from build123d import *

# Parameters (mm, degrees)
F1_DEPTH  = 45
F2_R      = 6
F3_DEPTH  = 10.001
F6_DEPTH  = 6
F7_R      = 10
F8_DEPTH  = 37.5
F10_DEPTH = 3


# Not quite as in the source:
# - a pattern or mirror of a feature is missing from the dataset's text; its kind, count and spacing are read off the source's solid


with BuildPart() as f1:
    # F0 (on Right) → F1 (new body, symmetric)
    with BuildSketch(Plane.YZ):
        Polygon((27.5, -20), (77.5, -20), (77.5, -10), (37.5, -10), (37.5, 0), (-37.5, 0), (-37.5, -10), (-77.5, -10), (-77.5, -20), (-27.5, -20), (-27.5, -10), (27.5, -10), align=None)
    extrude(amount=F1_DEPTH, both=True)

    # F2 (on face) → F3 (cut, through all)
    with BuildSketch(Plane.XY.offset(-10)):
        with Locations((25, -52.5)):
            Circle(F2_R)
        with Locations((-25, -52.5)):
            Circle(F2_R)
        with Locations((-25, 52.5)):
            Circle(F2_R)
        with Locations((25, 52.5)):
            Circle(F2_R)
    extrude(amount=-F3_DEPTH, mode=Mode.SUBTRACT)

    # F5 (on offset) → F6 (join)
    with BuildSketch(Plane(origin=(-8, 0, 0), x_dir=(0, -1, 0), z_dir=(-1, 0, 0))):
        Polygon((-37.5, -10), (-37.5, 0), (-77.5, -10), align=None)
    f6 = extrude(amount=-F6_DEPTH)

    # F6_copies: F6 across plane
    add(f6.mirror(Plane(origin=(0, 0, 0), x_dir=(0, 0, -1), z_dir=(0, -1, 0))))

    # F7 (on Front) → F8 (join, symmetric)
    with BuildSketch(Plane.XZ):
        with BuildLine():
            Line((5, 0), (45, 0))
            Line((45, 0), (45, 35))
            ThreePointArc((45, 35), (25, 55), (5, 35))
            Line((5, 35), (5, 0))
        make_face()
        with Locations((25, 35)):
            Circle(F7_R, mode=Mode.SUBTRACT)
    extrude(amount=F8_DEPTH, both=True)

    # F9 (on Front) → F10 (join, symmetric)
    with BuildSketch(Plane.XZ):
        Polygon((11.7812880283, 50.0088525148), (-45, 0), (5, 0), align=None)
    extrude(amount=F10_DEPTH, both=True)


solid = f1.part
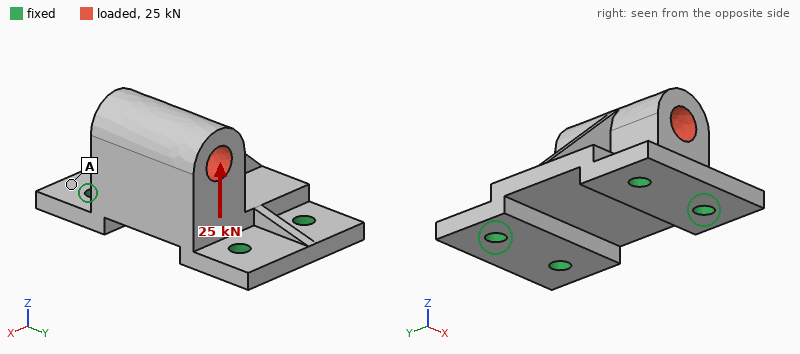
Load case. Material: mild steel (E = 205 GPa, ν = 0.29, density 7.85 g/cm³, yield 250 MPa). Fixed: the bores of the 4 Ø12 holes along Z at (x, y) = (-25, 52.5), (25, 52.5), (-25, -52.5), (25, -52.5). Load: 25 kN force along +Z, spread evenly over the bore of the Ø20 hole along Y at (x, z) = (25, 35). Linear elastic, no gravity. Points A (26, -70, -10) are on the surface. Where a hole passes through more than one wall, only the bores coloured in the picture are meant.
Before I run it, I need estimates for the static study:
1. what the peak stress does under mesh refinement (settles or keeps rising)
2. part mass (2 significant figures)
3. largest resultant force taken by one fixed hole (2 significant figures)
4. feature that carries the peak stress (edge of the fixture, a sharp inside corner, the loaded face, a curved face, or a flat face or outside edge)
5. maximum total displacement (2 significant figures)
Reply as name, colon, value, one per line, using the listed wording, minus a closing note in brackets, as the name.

what the peak stress does under mesh refinement: keeps rising
part mass: 2.3 kg
largest resultant force taken by one fixed hole: 14 kN
feature that carries the peak stress: edge of the fixture
maximum total displacement: 34 µm
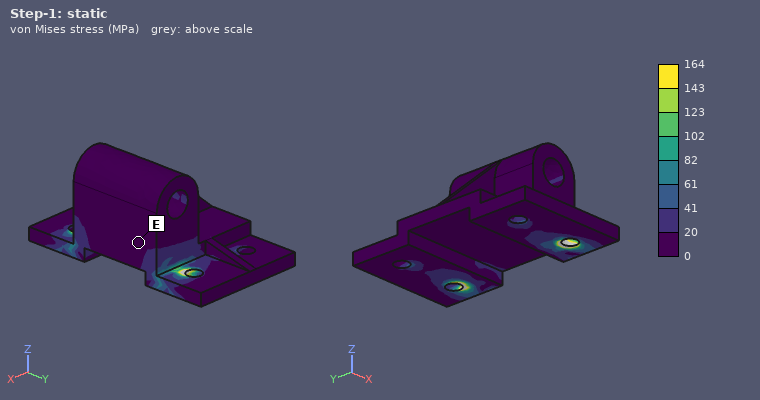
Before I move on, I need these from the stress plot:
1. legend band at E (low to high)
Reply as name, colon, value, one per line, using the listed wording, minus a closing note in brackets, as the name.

legend band at E: 0 to 20 MPa
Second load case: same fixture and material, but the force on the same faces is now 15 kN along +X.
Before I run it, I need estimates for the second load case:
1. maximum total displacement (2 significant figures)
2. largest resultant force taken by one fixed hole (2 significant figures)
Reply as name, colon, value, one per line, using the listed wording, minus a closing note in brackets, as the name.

maximum total displacement: 68 µm
largest resultant force taken by one fixed hole: 12 kN
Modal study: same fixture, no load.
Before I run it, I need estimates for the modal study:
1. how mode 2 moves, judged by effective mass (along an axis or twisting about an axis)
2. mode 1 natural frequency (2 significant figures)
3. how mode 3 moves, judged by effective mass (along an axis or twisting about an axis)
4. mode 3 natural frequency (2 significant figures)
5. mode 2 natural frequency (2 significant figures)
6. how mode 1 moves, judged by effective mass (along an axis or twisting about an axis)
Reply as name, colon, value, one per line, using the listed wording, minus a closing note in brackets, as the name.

how mode 2 moves, judged by effective mass: along Y
mode 1 natural frequency: 2900 Hz
how mode 3 moves, judged by effective mass: along Z
mode 3 natural frequency: 5300 Hz
mode 2 natural frequency: 5100 Hz
how mode 1 moves, judged by effective mass: along X
